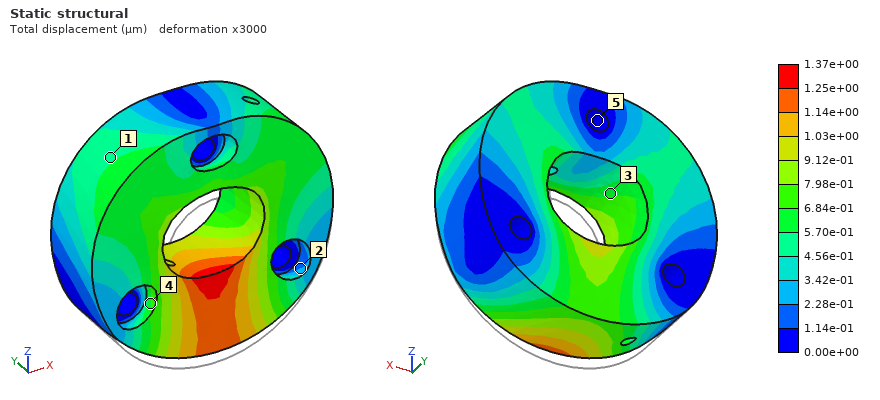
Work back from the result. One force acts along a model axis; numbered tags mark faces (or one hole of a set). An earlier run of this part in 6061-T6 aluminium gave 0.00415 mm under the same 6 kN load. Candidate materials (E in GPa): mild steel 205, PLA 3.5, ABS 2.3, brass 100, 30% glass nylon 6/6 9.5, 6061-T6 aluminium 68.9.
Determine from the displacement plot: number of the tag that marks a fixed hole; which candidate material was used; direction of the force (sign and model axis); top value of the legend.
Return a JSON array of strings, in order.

["5", "mild steel", "+Z", "1.37e+00 µm"]
